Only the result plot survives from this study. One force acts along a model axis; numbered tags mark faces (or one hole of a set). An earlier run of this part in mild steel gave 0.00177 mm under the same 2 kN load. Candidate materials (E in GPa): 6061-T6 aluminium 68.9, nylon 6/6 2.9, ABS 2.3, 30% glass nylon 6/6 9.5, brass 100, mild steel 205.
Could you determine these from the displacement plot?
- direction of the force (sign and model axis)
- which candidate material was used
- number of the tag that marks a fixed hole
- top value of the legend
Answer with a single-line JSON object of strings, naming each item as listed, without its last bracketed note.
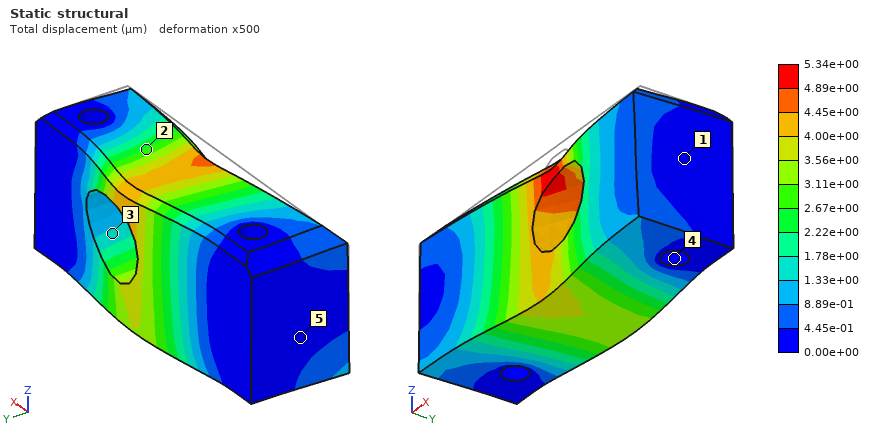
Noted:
{"direction of the force": "-Z", "which candidate material was used": "6061-T6 aluminium", "number of the tag that marks a fixed hole": "4", "top value of the legend": "5.34e+00 µm"}
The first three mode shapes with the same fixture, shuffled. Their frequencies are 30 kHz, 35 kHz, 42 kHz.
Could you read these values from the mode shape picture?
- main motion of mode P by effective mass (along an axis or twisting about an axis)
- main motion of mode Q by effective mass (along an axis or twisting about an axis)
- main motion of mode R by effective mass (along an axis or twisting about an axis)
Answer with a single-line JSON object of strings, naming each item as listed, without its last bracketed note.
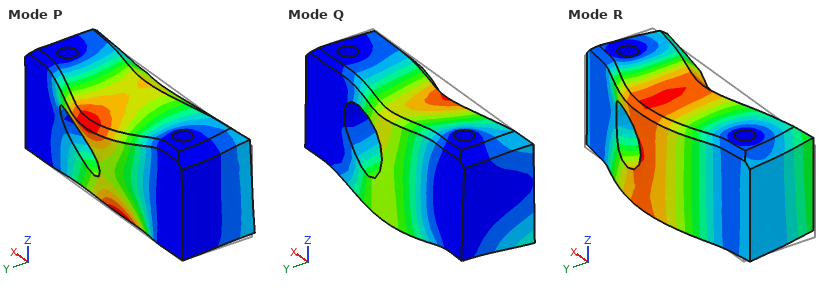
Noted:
{"main motion of mode P by effective mass": "twisting about X", "main motion of mode Q by effective mass": "along Z", "main motion of mode R by effective mass": "along Y"}
